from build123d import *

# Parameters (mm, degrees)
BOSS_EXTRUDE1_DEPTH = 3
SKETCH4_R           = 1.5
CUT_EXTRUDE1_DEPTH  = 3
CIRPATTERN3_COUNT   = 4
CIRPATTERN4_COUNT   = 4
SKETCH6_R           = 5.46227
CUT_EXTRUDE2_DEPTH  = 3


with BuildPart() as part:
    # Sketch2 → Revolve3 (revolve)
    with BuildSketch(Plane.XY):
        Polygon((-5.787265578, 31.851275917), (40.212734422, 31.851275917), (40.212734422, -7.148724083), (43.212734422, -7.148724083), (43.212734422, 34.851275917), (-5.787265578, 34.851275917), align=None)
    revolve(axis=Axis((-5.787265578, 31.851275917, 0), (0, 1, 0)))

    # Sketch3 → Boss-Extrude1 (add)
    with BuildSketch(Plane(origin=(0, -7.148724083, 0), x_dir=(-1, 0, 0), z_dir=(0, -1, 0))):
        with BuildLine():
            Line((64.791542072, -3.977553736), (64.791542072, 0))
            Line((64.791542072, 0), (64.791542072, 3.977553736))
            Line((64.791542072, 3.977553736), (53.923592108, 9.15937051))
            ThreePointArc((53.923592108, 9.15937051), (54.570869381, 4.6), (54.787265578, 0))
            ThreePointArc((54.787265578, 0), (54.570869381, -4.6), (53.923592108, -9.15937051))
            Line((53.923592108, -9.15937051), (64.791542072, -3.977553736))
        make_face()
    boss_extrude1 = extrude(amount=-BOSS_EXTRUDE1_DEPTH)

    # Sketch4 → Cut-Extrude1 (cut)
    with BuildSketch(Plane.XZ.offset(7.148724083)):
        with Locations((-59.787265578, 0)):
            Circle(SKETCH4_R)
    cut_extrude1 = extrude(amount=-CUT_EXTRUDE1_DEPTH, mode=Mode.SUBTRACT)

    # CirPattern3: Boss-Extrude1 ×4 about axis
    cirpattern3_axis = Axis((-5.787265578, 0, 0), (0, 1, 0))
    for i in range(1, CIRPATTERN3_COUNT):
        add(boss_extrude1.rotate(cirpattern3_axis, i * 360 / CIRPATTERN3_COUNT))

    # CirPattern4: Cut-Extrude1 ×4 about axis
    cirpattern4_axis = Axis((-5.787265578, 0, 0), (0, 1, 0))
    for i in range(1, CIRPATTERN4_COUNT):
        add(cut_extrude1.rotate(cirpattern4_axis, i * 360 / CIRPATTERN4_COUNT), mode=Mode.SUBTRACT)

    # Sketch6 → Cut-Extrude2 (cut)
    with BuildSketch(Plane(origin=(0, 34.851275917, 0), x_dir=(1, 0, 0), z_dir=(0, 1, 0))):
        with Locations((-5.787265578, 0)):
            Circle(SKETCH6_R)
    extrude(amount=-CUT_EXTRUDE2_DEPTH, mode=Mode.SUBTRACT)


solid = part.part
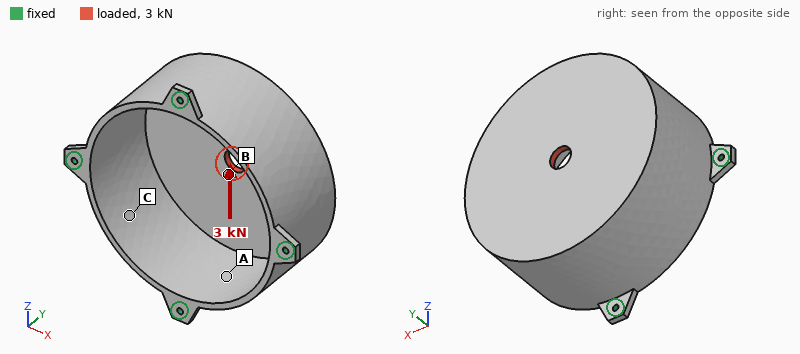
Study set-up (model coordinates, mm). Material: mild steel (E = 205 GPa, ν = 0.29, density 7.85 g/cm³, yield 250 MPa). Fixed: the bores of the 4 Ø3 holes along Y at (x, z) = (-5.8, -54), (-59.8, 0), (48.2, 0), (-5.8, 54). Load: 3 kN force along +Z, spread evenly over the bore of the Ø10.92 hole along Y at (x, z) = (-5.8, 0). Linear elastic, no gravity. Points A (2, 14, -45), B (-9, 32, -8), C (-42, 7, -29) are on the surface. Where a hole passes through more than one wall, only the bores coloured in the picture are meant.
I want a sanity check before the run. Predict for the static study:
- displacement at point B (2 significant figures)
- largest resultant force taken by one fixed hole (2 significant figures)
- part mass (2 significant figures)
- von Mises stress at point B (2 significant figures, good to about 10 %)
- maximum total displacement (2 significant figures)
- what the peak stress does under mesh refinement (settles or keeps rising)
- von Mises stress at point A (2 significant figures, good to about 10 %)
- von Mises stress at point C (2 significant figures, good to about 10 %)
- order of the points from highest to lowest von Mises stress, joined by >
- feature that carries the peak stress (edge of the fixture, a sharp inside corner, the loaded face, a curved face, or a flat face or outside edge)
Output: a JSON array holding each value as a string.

["20 µm", "1.3 kN", "460 g", "25 MPa", "22 µm", "keeps rising", "18 MPa", "8.1 MPa", "B > A > C", "edge of the fixture"]
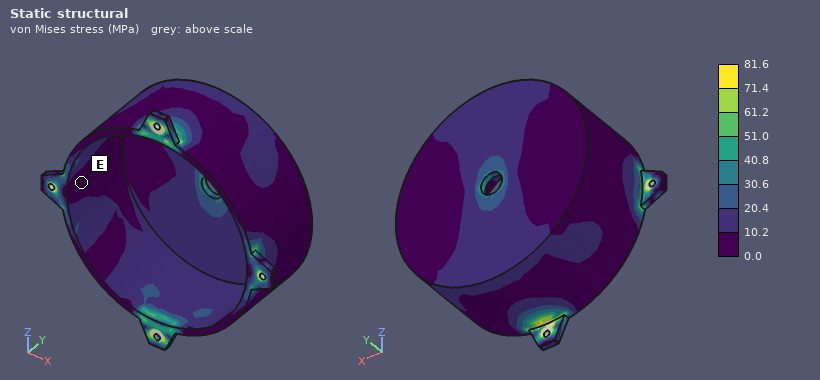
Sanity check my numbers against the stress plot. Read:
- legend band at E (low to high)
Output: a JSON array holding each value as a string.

["0.0 to 10.2 MPa"]
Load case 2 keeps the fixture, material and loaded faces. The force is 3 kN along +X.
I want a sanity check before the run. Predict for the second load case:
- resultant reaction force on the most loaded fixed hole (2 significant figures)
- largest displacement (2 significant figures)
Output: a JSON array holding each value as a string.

["1.3 kN", "22 µm"]
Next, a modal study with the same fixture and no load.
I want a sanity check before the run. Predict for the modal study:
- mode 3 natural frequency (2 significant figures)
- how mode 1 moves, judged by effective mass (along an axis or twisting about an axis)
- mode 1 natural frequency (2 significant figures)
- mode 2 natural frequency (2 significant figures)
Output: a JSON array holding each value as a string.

["3500 Hz", "along Y", "2800 Hz", "3500 Hz"]
